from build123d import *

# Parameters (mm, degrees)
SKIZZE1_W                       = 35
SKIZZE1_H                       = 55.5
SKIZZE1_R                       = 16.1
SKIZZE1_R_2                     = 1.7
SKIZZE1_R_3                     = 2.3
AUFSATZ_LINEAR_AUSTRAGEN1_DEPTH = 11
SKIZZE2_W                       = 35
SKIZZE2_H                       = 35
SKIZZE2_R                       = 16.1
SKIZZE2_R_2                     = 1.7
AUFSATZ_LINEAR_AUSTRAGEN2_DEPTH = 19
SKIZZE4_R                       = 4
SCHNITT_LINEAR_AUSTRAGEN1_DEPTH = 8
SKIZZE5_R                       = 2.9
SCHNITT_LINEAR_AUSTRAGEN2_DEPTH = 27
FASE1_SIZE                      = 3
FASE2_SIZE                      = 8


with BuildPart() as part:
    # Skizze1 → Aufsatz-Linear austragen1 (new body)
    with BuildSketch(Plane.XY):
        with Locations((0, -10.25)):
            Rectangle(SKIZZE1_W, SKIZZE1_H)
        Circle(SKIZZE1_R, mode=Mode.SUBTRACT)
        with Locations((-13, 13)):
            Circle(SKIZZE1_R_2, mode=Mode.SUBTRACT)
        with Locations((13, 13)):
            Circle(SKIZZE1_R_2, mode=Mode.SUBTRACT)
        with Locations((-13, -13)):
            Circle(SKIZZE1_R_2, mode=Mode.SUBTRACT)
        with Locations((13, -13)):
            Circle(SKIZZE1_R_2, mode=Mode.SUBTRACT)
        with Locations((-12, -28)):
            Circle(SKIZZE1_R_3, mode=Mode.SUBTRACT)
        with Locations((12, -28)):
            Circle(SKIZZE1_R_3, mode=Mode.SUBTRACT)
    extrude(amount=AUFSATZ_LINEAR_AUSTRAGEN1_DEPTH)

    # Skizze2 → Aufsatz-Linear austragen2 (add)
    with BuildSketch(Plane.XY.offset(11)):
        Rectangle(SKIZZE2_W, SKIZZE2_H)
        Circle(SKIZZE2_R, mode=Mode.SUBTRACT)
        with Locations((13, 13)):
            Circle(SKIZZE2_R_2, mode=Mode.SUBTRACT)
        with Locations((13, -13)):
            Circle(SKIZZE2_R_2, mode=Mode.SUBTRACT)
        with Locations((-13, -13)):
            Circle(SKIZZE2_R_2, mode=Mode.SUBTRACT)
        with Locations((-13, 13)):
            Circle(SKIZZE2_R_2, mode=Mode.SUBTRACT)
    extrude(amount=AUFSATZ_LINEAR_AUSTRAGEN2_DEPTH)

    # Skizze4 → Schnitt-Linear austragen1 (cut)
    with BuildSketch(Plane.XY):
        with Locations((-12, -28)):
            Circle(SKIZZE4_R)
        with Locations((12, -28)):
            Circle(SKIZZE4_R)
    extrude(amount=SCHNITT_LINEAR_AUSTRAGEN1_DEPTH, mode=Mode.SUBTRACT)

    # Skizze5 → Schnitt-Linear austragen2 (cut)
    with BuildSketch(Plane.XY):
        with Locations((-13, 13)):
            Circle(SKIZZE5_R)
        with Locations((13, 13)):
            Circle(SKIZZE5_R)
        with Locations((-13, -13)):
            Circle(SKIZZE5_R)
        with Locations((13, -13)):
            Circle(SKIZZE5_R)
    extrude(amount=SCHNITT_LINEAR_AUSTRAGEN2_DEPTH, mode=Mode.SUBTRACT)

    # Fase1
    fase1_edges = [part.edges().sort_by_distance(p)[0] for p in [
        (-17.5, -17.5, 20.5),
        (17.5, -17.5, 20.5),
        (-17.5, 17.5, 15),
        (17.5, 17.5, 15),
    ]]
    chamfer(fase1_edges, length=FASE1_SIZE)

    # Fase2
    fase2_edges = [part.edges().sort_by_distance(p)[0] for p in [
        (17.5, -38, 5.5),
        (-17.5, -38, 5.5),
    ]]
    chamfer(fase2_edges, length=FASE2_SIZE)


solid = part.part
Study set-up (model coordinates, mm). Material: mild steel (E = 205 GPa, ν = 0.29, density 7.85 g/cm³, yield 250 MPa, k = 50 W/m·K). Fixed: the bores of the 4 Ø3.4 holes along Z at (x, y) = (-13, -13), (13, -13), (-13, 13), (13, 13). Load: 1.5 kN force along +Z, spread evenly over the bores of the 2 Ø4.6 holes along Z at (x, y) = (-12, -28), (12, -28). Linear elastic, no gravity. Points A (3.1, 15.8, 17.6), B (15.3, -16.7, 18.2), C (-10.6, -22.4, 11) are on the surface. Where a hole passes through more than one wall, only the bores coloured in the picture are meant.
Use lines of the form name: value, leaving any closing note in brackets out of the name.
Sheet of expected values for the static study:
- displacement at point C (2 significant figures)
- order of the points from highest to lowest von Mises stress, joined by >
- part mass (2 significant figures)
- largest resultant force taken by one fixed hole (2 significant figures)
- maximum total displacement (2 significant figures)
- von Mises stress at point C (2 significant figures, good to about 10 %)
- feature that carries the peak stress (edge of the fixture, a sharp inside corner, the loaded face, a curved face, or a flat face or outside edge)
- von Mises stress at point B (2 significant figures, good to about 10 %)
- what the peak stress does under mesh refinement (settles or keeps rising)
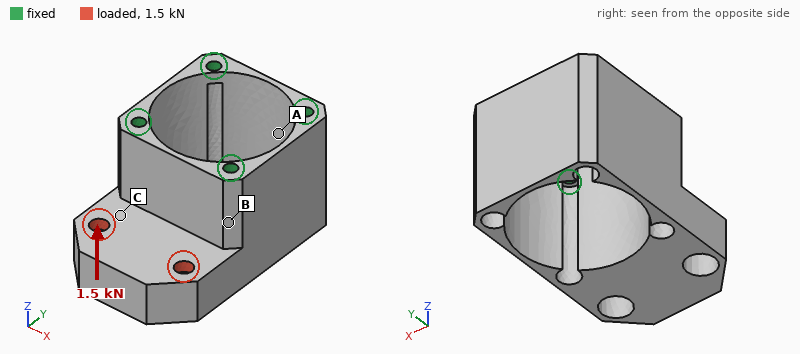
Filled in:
displacement at point C: 13 µm
order of the points from highest to lowest von Mises stress, joined by >: B > C > A
part mass: 120 g
largest resultant force taken by one fixed hole: 1.2 kN
maximum total displacement: 40 µm
von Mises stress at point C: 24 MPa
feature that carries the peak stress: a sharp inside corner
von Mises stress at point B: 39 MPa
what the peak stress does under mesh refinement: keeps rising
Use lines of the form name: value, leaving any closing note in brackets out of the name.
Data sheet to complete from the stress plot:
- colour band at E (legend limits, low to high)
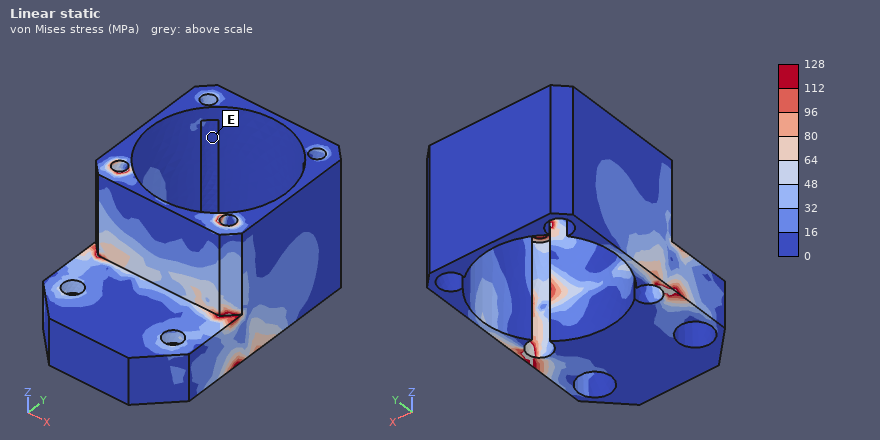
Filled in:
colour band at E: 0 to 16 MPa
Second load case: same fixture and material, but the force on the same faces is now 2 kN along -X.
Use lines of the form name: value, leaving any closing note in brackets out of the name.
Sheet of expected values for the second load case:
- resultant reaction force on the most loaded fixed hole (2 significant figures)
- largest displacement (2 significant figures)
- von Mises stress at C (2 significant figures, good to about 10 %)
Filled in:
resultant reaction force on the most loaded fixed hole: 1.4 kN
largest displacement: 19 µm
von Mises stress at C: 31 MPa
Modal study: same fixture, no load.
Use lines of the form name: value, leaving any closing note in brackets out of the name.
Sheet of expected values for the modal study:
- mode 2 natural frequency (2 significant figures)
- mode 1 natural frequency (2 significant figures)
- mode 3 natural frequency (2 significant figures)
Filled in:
mode 2 natural frequency: 6600 Hz
mode 1 natural frequency: 5300 Hz
mode 3 natural frequency: 6700 Hz
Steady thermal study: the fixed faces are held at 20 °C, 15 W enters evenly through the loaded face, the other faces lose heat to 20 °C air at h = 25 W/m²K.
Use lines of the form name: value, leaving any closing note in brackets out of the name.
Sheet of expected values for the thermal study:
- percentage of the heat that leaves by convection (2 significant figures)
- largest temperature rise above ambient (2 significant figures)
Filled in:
percentage of the heat that leaves by convection: 34 %
largest temperature rise above ambient: 55 K
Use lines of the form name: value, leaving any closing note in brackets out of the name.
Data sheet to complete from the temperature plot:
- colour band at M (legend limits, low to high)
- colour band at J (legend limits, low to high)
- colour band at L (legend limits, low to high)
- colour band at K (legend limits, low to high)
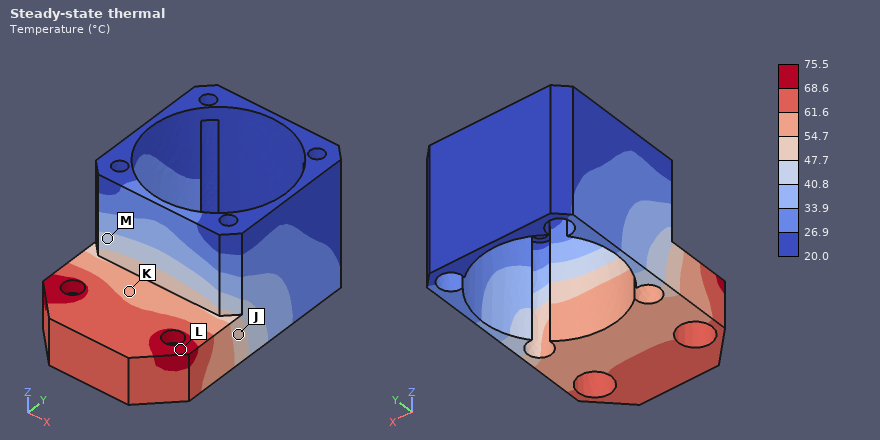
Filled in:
colour band at M: 40.8 to 47.7 °C
colour band at J: 47.7 to 54.7 °C
colour band at L: 68.6 to 75.5 °C
colour band at K: 54.7 to 61.6 °C
